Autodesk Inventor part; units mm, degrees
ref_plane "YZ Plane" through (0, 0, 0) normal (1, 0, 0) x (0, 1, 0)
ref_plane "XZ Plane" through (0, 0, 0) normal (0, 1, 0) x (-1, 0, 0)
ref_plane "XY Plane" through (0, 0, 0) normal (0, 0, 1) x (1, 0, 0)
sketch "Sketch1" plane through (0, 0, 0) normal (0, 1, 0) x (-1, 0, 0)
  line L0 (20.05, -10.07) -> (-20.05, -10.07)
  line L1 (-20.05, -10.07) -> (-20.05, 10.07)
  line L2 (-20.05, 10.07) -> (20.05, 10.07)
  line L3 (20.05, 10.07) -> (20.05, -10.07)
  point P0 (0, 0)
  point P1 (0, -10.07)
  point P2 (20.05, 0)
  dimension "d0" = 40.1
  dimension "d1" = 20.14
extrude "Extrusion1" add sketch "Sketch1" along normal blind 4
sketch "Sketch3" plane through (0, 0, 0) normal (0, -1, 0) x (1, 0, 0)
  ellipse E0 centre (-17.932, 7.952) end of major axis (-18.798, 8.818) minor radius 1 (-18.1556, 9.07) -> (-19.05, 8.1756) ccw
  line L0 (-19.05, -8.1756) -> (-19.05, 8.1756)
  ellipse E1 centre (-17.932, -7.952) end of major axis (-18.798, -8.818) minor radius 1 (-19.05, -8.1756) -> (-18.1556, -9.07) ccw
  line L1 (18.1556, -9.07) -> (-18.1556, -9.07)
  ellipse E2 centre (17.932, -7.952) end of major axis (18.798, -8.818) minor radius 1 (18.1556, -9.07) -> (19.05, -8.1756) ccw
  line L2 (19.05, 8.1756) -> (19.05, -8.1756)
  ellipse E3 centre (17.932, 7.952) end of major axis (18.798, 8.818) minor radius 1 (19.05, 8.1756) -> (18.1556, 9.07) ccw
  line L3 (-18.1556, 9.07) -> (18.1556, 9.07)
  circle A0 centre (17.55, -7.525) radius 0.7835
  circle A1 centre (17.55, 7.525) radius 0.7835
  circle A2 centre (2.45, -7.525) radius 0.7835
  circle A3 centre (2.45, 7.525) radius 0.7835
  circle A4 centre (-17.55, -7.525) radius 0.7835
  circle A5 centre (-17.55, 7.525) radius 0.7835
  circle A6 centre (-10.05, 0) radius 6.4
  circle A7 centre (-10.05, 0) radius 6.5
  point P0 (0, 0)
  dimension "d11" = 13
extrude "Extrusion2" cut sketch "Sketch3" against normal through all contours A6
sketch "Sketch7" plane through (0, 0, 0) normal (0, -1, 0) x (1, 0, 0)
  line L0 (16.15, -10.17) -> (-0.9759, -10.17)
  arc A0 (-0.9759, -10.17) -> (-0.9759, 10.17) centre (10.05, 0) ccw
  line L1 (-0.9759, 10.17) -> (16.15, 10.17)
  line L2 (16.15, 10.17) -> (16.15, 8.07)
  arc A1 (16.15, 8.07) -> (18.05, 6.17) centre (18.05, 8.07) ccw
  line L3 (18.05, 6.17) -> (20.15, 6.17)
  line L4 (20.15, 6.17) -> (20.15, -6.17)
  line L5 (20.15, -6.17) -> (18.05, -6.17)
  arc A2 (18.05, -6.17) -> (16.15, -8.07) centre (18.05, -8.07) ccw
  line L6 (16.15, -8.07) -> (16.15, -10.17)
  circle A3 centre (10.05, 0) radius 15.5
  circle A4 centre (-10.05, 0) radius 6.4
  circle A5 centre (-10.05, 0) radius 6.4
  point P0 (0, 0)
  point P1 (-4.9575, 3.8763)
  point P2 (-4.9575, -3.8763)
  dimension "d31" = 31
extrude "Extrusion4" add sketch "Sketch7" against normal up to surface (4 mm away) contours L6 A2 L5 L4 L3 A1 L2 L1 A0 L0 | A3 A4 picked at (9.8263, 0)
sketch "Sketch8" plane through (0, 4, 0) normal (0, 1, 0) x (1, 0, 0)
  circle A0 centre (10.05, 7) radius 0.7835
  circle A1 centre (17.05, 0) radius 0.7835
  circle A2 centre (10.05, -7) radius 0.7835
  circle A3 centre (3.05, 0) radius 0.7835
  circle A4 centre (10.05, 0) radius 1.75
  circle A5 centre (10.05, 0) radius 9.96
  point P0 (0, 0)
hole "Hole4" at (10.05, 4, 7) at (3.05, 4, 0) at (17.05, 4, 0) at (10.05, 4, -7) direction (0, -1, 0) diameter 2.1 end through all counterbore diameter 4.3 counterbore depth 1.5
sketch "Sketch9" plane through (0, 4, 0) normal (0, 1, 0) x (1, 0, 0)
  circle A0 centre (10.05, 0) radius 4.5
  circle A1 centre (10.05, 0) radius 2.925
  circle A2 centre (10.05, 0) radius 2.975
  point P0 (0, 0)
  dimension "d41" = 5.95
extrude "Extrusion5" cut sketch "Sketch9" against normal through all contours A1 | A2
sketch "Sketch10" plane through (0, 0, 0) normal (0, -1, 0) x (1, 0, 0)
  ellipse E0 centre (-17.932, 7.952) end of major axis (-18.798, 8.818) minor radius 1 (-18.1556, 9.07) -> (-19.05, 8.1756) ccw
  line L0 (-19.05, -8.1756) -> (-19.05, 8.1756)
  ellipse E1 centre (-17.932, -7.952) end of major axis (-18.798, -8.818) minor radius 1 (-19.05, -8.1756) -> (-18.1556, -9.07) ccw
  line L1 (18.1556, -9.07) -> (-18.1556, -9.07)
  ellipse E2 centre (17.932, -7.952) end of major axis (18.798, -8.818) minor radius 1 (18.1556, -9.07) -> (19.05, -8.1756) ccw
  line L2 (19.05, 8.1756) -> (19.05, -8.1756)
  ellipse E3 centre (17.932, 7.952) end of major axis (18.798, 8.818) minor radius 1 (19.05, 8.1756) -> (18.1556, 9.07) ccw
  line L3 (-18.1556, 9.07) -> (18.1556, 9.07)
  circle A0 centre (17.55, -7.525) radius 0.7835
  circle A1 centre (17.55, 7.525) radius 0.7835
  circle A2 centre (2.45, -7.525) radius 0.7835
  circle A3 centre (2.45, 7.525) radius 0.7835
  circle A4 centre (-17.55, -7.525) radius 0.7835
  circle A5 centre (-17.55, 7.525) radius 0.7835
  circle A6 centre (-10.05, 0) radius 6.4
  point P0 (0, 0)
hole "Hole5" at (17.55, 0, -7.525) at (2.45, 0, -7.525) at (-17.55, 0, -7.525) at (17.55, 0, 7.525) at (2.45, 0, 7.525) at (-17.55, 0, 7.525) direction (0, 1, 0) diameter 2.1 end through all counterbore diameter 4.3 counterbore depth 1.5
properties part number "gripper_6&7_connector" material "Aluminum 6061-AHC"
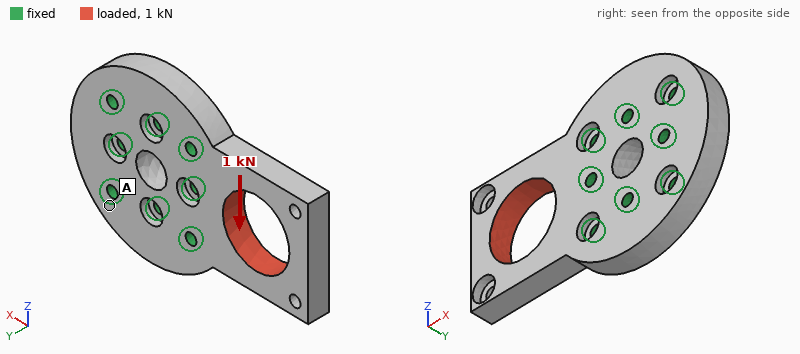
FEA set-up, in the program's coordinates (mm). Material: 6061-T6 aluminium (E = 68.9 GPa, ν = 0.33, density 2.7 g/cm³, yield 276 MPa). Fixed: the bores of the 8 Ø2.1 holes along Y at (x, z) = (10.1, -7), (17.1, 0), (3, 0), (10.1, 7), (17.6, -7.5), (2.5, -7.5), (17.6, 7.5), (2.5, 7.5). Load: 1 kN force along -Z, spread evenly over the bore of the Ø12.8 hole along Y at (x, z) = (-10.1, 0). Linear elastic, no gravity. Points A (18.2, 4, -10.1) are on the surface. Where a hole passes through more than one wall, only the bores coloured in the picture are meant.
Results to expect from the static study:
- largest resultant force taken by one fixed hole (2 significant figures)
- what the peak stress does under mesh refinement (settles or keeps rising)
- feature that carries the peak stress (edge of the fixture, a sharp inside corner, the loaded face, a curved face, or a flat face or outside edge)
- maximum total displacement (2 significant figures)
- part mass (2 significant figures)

600 N
keeps rising
edge of the fixture
52 µm
9.1 g
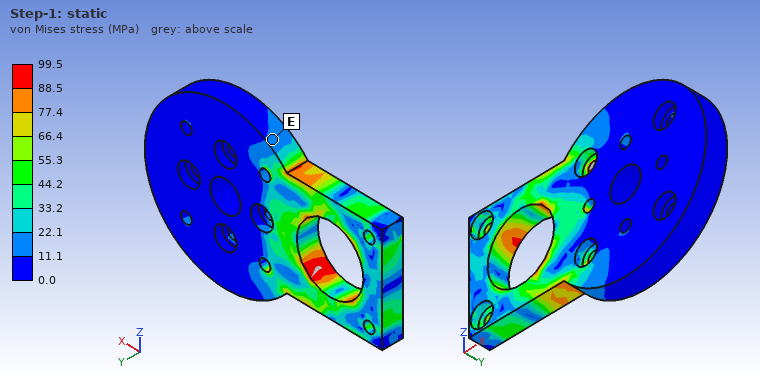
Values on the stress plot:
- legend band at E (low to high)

11.1 to 22.1 MPa
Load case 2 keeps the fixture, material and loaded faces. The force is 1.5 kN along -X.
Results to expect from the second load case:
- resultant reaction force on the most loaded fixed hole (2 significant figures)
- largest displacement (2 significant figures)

480 N
18 µm
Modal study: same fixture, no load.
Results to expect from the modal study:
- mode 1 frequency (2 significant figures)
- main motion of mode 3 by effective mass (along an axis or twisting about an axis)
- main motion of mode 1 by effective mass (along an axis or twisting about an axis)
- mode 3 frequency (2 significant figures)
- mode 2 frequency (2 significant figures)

5900 Hz
along Z
along Y
16 kHz
13 kHz
